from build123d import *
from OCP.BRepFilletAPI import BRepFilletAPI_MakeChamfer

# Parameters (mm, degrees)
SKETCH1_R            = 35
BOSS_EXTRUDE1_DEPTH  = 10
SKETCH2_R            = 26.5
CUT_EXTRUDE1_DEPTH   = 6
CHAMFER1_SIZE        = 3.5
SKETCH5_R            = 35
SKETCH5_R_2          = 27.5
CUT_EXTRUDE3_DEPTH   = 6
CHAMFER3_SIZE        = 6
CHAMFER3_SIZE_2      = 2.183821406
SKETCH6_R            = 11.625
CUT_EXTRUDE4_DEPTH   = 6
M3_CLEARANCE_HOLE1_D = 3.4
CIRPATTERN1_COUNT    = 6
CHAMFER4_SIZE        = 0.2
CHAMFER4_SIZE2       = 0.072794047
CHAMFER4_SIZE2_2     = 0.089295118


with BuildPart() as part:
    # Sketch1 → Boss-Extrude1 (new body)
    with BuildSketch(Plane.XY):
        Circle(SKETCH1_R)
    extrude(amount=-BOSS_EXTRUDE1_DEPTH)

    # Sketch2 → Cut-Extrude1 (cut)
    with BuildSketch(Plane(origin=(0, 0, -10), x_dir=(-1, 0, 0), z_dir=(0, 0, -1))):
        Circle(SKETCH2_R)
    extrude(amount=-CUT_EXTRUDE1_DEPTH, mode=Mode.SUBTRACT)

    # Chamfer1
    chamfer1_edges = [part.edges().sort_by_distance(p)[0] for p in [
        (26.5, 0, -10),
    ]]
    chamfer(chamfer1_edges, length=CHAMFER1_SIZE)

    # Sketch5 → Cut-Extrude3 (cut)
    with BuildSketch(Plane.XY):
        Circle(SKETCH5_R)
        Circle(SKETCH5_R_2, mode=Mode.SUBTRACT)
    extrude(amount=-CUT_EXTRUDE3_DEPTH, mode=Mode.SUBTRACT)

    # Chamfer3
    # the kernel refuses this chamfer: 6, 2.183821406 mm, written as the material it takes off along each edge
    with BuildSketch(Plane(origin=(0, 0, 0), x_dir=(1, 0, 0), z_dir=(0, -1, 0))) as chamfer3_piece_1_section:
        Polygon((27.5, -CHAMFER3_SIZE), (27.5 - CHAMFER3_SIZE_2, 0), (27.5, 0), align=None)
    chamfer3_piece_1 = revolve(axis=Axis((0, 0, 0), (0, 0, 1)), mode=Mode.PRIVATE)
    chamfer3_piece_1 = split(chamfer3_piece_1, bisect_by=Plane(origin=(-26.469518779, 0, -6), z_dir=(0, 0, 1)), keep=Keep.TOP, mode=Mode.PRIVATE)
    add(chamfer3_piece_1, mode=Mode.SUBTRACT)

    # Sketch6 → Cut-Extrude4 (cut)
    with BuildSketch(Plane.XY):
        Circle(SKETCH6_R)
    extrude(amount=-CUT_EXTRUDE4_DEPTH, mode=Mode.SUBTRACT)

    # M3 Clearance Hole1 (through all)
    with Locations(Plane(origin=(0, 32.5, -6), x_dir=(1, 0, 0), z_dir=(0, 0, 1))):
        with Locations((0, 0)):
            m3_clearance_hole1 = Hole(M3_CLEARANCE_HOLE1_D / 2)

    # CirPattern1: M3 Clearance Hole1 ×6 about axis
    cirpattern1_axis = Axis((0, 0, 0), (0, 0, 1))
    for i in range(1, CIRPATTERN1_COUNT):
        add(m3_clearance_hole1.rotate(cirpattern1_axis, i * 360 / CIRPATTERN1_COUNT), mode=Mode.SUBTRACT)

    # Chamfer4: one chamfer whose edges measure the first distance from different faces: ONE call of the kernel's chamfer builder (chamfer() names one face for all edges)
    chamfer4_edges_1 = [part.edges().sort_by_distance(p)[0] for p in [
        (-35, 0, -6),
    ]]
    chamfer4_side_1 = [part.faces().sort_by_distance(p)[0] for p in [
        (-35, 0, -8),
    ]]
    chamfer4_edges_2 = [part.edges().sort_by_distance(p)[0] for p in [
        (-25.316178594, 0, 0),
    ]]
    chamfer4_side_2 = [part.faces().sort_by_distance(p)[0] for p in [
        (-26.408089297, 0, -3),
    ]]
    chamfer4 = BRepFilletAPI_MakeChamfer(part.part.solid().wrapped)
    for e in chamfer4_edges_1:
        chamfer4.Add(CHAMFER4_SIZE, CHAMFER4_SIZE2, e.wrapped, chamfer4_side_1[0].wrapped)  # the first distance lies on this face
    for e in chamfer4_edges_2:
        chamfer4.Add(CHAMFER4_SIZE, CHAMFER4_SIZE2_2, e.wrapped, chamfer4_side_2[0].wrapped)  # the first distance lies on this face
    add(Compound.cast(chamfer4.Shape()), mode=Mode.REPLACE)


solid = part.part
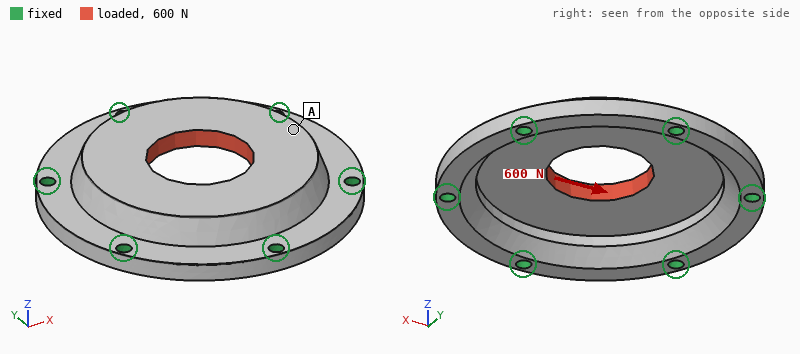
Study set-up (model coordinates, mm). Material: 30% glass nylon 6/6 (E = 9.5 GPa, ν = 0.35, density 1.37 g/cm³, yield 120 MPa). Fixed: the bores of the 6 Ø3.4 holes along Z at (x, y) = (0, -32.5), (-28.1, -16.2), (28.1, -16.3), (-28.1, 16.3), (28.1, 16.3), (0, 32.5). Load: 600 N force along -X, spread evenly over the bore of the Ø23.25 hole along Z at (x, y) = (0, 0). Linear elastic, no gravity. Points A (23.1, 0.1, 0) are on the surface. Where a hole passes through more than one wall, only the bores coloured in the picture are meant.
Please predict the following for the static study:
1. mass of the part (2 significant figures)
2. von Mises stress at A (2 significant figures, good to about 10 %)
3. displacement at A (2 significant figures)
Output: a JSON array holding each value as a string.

["17 g", "3.3 MPa", "22 µm"]
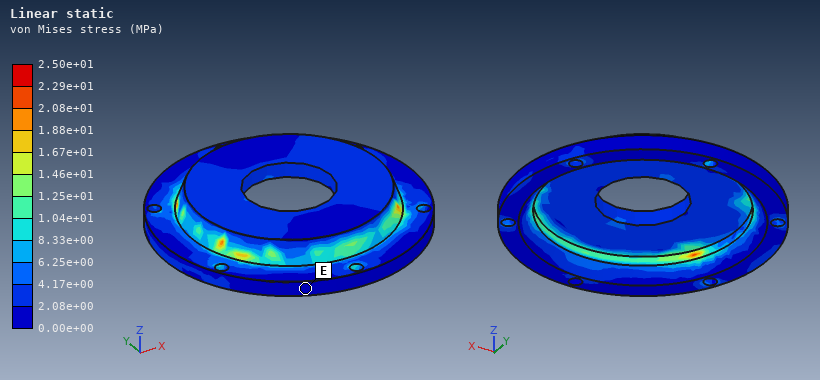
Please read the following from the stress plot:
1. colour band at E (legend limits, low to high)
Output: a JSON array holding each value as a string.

["0.00e+00 to 2.08e+00 MPa"]
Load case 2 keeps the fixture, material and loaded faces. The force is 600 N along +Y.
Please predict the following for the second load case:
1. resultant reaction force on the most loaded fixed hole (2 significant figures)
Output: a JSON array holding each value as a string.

["120 N"]
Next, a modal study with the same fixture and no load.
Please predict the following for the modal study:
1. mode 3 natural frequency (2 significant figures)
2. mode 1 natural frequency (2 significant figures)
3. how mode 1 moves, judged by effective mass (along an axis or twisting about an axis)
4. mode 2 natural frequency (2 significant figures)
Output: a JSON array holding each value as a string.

["7300 Hz", "4300 Hz", "along Z", "7200 Hz"]
